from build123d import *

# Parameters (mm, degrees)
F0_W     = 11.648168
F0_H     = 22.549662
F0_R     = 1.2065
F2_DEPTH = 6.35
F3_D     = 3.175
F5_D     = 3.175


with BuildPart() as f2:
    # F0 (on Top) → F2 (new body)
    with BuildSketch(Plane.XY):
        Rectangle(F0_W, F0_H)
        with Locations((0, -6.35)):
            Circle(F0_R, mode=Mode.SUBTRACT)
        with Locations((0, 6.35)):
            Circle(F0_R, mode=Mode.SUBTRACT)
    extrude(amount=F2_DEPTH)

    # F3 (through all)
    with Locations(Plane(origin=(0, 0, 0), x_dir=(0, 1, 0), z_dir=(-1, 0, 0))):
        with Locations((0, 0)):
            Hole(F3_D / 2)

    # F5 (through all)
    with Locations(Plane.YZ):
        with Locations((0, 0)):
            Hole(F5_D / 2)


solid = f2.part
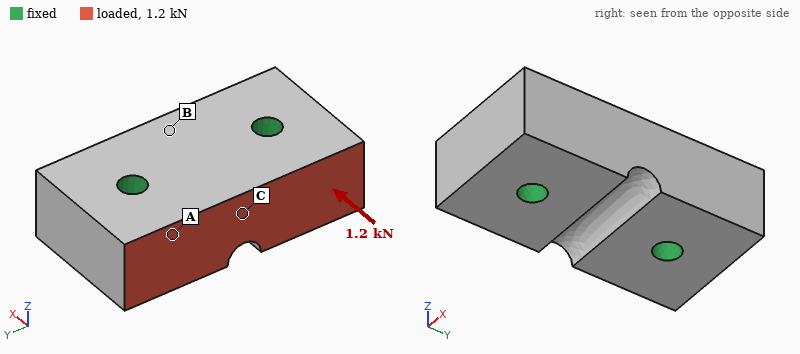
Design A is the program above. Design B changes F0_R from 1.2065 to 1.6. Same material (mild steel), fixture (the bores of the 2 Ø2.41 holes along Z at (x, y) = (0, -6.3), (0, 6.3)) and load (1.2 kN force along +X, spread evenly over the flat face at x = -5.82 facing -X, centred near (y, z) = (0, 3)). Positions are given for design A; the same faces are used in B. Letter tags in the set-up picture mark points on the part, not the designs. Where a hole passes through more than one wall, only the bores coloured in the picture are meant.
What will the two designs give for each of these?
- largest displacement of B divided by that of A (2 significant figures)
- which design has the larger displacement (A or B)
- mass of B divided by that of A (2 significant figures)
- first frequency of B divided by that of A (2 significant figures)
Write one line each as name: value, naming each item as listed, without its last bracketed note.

largest displacement of B divided by that of A: 0.90
which design has the larger displacement: A
mass of B divided by that of A: 0.97
first frequency of B divided by that of A: 1.2
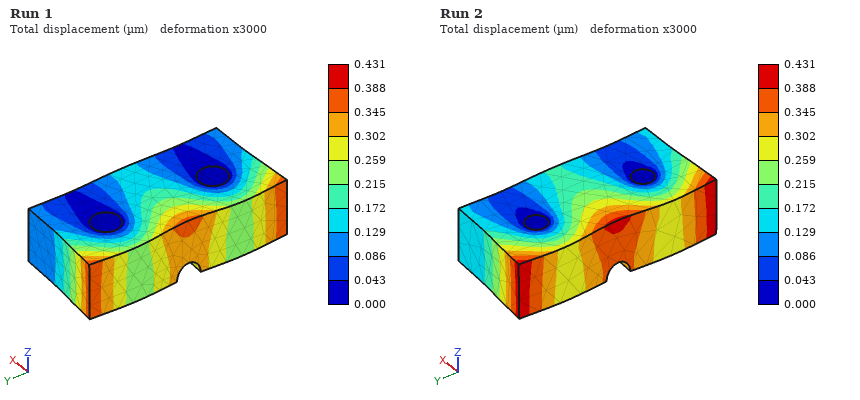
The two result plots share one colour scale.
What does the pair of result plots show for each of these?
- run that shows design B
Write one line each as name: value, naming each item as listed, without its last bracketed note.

run that shows design B: Run 1
